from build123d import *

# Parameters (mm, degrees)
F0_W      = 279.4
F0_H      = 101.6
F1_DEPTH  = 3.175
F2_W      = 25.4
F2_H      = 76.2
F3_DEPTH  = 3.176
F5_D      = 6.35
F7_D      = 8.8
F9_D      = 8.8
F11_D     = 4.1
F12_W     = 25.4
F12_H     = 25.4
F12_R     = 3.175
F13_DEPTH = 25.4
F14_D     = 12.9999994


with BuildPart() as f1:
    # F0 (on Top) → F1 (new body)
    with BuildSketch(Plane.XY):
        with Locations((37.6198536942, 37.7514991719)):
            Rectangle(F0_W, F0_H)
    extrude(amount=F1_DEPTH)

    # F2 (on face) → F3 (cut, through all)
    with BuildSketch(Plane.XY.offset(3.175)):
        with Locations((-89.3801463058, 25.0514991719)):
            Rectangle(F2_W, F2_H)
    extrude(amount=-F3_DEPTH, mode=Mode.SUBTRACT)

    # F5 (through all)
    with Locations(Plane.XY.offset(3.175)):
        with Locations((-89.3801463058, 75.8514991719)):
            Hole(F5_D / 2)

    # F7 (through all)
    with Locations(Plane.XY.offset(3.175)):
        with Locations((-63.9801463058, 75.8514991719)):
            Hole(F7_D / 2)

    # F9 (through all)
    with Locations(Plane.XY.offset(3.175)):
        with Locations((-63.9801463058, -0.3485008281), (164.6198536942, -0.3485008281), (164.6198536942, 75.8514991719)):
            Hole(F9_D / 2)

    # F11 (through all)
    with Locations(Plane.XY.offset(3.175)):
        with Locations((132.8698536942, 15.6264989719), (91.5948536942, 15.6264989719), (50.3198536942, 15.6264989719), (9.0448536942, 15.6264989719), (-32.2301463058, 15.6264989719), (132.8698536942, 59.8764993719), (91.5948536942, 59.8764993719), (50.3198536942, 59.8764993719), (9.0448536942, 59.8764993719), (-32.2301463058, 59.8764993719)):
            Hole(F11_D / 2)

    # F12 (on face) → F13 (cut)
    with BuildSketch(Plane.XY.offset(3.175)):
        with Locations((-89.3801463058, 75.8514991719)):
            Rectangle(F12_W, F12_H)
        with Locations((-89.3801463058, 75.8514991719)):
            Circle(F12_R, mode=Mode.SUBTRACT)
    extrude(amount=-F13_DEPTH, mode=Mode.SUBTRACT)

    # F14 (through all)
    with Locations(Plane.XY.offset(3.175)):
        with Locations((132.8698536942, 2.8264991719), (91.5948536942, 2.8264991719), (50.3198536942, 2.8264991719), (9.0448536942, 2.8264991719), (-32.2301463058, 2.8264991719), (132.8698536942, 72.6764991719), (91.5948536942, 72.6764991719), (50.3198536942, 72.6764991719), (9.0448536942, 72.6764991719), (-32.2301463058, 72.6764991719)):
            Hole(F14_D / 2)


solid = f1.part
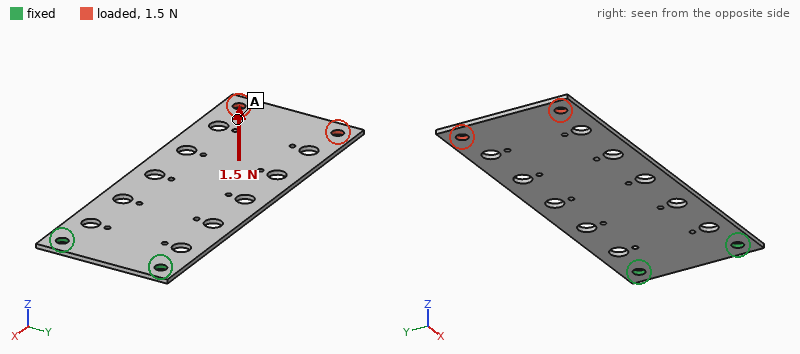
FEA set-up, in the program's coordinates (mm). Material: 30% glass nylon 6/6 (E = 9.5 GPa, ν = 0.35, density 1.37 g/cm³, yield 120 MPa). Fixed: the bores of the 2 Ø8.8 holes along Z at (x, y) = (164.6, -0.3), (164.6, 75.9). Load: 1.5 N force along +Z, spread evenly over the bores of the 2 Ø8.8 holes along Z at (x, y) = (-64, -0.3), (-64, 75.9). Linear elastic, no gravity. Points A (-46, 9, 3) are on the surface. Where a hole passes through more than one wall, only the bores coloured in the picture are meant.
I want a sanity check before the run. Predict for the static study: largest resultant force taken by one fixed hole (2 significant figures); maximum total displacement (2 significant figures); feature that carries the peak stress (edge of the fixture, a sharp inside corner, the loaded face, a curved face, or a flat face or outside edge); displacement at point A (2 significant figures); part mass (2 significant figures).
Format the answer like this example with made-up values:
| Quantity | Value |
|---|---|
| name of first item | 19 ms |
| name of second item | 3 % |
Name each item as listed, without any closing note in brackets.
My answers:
| Quantity | Value |
|---|---|
| largest resultant force taken by one fixed hole | 0.75 N |
| maximum total displacement | 2.9 mm |
| feature that carries the peak stress | a curved face |
| displacement at point A | 2.3 mm |
| part mass | 100 g |
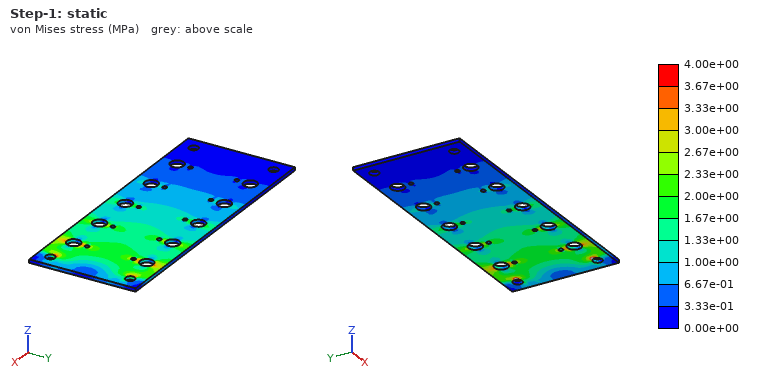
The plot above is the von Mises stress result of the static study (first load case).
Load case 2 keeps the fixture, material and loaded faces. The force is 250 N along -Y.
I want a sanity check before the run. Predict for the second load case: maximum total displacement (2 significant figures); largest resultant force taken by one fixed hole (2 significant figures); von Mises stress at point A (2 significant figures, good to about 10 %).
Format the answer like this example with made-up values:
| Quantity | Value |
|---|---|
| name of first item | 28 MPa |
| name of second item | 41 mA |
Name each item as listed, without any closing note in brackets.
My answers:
| Quantity | Value |
|---|---|
| maximum total displacement | 0.63 mm |
| largest resultant force taken by one fixed hole | 730 N |
| von Mises stress at point A | 1.4 MPa |
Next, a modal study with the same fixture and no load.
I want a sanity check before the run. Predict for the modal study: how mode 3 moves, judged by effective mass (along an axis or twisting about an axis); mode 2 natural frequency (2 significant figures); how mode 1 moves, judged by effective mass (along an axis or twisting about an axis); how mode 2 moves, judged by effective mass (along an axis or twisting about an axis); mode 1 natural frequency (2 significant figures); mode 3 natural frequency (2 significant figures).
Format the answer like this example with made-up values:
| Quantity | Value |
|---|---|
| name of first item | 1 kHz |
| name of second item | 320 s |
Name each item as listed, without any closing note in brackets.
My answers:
| Quantity | Value |
|---|---|
| how mode 3 moves, judged by effective mass | along Z |
| mode 2 natural frequency | 120 Hz |
| how mode 1 moves, judged by effective mass | along Z |
| how mode 2 moves, judged by effective mass | twisting about X |
| mode 1 natural frequency | 22 Hz |
| mode 3 natural frequency | 140 Hz |
